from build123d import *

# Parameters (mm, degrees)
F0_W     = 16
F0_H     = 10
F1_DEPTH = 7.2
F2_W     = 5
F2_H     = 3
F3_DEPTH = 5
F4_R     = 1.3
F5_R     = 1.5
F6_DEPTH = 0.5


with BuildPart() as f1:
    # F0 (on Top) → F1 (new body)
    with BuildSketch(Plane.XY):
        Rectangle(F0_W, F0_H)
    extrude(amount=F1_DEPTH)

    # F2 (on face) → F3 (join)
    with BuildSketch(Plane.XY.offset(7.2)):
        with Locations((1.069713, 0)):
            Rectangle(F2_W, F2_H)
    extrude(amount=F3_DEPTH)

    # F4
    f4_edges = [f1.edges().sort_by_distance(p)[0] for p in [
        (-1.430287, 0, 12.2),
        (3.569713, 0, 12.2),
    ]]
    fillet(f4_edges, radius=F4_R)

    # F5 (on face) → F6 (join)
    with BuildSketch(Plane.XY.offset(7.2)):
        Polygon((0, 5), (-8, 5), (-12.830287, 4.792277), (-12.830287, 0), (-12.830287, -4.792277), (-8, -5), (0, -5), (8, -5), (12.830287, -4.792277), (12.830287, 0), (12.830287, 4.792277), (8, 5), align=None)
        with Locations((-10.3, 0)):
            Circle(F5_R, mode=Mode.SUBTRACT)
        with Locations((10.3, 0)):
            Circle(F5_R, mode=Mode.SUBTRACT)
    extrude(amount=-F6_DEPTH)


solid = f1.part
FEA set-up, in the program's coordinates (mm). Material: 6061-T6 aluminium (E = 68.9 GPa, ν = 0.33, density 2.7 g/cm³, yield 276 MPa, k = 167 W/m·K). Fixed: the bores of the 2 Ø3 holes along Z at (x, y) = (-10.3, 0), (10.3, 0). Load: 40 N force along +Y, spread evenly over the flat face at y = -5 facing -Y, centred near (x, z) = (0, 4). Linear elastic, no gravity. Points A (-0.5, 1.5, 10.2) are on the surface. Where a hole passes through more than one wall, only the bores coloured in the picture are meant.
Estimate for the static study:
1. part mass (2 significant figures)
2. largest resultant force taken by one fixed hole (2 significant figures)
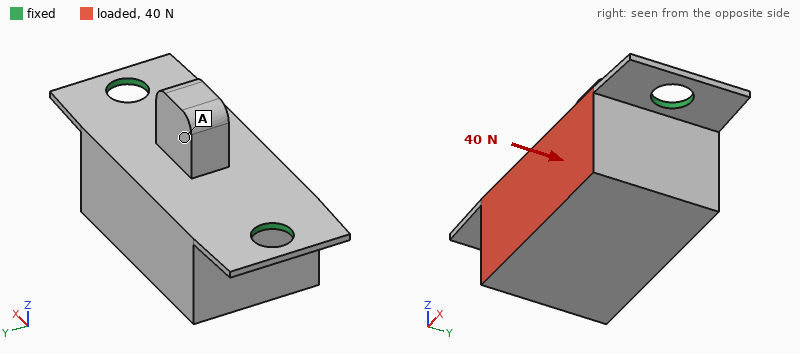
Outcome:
3.4 g
20 N
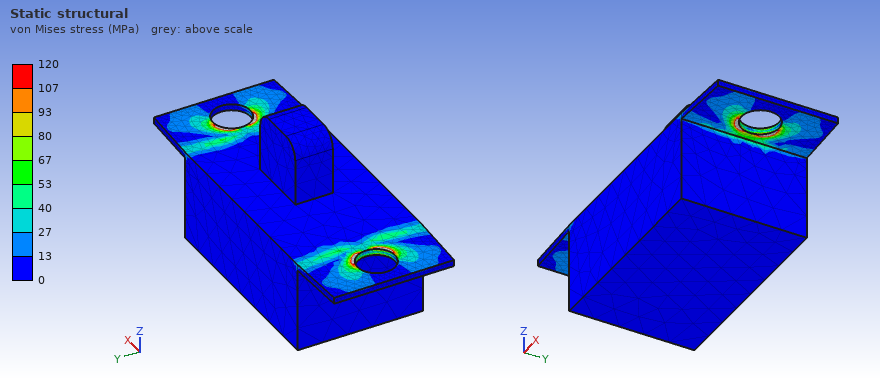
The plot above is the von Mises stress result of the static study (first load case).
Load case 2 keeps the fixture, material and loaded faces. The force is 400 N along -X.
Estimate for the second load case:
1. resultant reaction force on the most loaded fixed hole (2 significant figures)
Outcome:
240 N
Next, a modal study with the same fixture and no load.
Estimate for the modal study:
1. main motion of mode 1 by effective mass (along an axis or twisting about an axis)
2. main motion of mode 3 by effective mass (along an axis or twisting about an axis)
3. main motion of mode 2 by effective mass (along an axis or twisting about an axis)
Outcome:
along Y
along X
along Z
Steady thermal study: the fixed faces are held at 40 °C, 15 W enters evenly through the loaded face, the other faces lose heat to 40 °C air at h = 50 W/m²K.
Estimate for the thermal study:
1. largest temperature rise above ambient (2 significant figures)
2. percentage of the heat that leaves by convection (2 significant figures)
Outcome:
28 K
5.7 %
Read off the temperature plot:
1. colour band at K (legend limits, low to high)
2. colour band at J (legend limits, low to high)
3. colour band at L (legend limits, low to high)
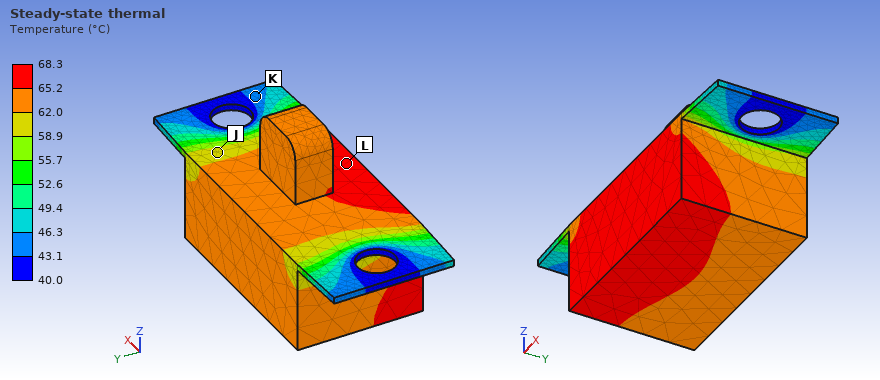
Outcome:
43.1 to 46.3 °C
58.9 to 62.0 °C
65.2 to 68.3 °C
